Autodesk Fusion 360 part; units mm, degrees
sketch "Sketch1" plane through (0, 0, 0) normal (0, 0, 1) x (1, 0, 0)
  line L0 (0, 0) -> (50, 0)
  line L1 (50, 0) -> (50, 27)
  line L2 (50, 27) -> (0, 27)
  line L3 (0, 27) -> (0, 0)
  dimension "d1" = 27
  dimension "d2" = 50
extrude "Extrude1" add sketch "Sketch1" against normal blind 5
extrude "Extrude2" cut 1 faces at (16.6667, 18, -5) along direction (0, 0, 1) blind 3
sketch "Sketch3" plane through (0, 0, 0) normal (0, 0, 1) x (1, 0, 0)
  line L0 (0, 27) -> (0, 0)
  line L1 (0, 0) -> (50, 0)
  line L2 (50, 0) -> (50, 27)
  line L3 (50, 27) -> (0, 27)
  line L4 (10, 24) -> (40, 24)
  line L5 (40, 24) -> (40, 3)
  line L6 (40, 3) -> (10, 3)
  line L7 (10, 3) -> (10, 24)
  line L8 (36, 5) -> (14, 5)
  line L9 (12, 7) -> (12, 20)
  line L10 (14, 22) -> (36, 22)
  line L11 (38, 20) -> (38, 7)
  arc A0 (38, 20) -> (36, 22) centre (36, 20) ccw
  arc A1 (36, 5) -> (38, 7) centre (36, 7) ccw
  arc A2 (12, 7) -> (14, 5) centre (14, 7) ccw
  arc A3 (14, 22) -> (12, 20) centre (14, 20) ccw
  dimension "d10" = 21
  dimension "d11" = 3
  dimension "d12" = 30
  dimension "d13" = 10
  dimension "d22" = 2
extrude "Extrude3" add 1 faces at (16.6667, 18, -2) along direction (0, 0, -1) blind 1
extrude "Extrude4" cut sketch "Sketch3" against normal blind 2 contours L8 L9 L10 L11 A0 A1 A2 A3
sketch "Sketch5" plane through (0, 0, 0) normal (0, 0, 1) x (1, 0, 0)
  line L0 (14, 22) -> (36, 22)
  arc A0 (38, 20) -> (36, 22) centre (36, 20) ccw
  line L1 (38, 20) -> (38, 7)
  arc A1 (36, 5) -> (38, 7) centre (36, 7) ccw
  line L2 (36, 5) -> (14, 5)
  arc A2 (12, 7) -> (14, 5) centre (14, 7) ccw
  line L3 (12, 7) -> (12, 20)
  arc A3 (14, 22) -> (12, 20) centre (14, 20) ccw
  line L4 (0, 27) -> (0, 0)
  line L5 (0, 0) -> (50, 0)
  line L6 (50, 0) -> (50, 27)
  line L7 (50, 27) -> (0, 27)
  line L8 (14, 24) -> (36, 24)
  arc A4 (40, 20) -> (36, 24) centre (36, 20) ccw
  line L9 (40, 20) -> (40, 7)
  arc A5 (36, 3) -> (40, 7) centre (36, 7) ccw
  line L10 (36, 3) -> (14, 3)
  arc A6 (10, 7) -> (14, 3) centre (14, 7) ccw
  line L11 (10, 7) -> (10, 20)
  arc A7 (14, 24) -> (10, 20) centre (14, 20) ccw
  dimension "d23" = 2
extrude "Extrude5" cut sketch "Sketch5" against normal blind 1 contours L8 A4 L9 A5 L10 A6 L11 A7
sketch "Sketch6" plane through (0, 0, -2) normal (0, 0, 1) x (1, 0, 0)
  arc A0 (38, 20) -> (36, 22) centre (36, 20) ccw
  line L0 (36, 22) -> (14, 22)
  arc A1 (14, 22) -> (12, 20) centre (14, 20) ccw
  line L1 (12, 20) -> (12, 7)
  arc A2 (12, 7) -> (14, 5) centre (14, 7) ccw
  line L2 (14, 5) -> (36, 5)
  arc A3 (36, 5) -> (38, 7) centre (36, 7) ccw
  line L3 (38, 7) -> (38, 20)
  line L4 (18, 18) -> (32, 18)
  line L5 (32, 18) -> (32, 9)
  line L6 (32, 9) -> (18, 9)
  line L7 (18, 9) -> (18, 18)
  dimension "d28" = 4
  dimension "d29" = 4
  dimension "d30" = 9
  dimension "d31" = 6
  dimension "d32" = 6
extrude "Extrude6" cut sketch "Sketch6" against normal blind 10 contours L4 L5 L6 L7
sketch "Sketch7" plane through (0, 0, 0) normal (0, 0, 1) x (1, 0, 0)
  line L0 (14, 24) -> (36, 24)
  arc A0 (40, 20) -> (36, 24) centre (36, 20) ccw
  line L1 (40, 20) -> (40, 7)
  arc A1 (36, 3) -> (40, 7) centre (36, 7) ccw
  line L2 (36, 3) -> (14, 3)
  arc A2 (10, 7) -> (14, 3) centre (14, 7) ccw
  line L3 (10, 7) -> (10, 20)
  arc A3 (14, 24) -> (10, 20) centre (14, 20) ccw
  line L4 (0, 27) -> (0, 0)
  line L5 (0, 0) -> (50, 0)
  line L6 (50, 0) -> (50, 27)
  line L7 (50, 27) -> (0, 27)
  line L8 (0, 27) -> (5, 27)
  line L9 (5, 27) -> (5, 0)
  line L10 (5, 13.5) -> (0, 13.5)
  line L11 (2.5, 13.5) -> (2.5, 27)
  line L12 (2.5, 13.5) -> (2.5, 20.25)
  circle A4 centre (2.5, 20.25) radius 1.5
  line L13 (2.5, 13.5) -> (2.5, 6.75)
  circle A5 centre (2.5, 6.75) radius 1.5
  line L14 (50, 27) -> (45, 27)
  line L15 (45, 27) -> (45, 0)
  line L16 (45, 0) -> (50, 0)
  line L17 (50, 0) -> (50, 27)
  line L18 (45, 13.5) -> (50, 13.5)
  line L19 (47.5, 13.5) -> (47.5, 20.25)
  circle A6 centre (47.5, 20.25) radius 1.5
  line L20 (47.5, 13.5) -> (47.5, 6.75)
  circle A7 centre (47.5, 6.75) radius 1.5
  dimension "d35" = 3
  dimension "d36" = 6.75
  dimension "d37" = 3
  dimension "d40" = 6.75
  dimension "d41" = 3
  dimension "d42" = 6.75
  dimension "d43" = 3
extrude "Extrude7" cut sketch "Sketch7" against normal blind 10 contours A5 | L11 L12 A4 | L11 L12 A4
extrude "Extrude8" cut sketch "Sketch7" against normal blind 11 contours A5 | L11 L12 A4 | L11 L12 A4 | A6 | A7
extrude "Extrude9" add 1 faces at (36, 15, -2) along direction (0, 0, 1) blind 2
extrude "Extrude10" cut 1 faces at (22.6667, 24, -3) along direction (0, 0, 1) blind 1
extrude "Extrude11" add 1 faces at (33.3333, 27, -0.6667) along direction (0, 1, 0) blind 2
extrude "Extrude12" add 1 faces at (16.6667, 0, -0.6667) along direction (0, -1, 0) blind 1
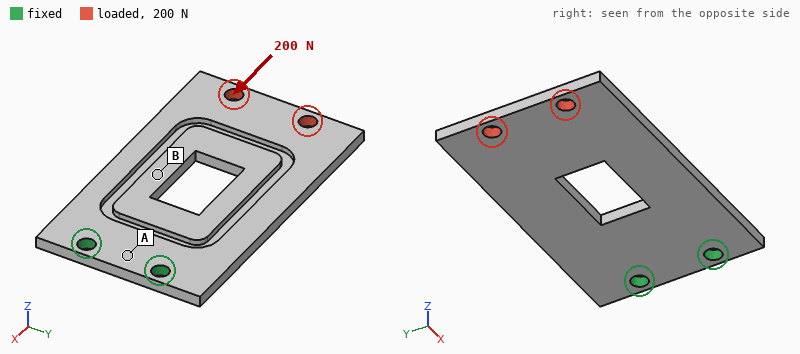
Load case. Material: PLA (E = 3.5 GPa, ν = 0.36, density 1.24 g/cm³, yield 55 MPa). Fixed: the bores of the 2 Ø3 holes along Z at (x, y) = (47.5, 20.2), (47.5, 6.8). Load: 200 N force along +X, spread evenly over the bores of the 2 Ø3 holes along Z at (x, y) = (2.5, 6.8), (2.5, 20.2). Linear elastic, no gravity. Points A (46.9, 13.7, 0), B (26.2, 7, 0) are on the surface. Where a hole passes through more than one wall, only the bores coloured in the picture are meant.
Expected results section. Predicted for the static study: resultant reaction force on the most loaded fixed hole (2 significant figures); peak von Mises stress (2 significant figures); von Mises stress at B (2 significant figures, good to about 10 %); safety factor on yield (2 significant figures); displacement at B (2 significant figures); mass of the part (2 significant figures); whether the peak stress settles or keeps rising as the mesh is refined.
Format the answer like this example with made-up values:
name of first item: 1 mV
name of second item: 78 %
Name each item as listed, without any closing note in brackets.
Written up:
resultant reaction force on the most loaded fixed hole: 100 N
peak von Mises stress: 19 MPa
von Mises stress at B: 7.0 MPa
safety factor on yield: 3.0
displacement at B: 0.13 mm
mass of the part: 3.1 g
whether the peak stress settles or keeps rising as the mesh is refined: settles
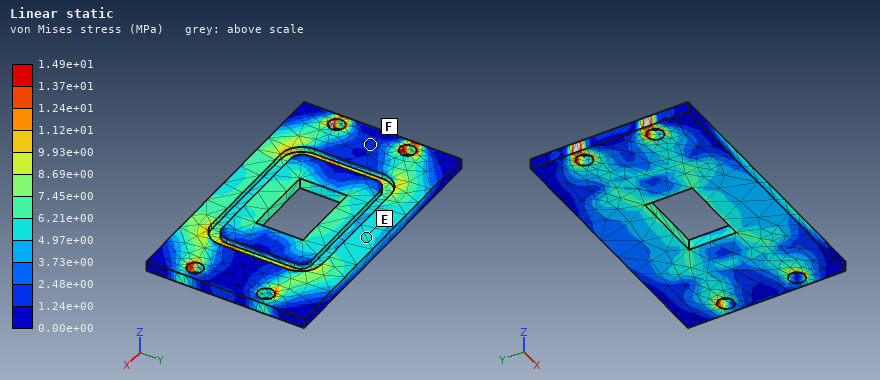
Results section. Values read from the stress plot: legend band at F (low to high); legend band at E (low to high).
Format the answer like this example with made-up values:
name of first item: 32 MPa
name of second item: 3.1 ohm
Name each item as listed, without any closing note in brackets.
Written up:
legend band at F: 1.24e+00 to 2.48e+00 MPa
legend band at E: 4.97e+00 to 6.21e+00 MPa
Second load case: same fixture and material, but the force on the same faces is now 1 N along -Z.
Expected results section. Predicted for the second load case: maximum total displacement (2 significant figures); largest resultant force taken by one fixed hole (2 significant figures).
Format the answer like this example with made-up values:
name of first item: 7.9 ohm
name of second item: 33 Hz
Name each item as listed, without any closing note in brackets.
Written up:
maximum total displacement: 0.68 mm
largest resultant force taken by one fixed hole: 1.6 N
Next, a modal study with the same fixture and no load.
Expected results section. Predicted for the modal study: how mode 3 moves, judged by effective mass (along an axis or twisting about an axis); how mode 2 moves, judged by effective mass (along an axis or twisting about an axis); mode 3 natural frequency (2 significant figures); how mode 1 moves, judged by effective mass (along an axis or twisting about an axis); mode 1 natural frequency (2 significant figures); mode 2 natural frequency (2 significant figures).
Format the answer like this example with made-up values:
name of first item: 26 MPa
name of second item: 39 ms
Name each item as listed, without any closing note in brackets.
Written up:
how mode 3 moves, judged by effective mass: along Z
how mode 2 moves, judged by effective mass: twisting about X
mode 3 natural frequency: 1400 Hz
how mode 1 moves, judged by effective mass: along Z
mode 1 natural frequency: 220 Hz
mode 2 natural frequency: 700 Hz
